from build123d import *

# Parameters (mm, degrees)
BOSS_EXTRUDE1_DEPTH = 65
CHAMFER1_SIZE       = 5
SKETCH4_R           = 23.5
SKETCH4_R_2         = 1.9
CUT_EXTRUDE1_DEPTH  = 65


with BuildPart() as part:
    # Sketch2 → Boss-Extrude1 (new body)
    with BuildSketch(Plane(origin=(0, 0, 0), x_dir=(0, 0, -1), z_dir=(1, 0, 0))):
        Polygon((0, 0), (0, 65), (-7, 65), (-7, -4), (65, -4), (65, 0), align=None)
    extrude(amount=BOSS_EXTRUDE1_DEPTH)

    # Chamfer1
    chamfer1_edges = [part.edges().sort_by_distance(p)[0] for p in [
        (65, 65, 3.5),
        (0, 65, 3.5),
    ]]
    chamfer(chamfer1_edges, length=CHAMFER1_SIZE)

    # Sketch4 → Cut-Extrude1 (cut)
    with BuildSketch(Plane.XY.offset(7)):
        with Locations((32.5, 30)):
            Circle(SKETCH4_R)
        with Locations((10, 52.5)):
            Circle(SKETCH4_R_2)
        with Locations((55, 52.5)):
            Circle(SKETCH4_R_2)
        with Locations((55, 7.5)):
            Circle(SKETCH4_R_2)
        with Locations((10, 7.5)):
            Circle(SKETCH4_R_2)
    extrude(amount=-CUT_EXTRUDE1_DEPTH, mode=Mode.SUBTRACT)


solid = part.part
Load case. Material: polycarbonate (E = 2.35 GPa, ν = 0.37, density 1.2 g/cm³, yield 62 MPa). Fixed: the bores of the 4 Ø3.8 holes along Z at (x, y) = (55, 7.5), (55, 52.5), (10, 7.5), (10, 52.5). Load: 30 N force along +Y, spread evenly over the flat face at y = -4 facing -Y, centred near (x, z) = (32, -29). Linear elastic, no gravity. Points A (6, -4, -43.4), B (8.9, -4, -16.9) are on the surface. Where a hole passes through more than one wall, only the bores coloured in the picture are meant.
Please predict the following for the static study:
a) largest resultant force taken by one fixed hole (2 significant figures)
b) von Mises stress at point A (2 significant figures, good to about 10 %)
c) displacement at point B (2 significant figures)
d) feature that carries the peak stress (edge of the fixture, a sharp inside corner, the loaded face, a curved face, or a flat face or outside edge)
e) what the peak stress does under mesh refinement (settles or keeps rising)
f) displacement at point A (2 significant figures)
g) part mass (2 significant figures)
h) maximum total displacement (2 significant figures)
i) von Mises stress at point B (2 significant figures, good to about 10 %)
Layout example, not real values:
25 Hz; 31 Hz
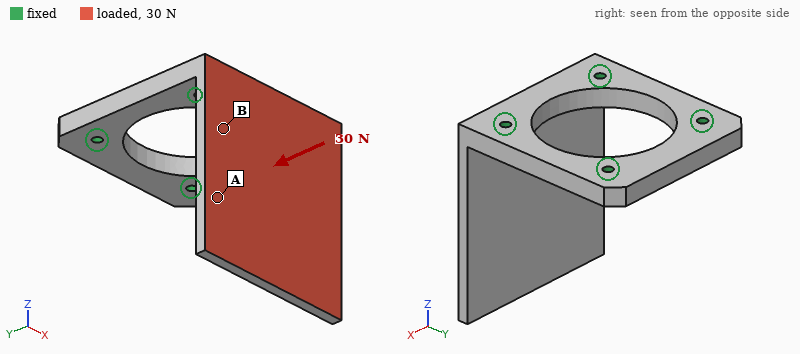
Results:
19 N; 0.64 MPa; 0.22 mm; edge of the fixture; keeps rising; 0.82 mm; 43 g; 1.4 mm; 2.7 MPa
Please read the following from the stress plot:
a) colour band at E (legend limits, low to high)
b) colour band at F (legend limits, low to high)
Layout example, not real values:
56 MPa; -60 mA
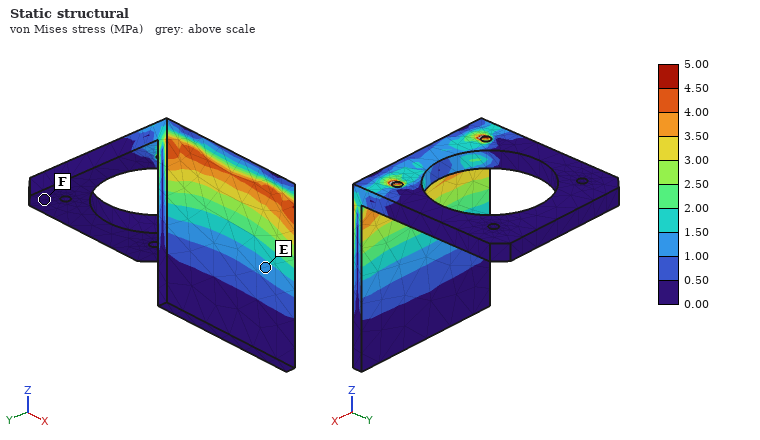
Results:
1.00 to 1.50 MPa; 0.00 to 0.50 MPa
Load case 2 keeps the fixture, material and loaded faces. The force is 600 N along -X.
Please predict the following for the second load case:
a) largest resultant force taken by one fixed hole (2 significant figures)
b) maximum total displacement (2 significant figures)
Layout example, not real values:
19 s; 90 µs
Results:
520 N; 0.72 mm
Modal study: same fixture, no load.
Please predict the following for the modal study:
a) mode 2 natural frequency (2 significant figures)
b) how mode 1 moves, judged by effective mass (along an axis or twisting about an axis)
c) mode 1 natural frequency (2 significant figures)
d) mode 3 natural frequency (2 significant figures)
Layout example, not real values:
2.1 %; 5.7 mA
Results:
490 Hz; along Y; 190 Hz; 1200 Hz
